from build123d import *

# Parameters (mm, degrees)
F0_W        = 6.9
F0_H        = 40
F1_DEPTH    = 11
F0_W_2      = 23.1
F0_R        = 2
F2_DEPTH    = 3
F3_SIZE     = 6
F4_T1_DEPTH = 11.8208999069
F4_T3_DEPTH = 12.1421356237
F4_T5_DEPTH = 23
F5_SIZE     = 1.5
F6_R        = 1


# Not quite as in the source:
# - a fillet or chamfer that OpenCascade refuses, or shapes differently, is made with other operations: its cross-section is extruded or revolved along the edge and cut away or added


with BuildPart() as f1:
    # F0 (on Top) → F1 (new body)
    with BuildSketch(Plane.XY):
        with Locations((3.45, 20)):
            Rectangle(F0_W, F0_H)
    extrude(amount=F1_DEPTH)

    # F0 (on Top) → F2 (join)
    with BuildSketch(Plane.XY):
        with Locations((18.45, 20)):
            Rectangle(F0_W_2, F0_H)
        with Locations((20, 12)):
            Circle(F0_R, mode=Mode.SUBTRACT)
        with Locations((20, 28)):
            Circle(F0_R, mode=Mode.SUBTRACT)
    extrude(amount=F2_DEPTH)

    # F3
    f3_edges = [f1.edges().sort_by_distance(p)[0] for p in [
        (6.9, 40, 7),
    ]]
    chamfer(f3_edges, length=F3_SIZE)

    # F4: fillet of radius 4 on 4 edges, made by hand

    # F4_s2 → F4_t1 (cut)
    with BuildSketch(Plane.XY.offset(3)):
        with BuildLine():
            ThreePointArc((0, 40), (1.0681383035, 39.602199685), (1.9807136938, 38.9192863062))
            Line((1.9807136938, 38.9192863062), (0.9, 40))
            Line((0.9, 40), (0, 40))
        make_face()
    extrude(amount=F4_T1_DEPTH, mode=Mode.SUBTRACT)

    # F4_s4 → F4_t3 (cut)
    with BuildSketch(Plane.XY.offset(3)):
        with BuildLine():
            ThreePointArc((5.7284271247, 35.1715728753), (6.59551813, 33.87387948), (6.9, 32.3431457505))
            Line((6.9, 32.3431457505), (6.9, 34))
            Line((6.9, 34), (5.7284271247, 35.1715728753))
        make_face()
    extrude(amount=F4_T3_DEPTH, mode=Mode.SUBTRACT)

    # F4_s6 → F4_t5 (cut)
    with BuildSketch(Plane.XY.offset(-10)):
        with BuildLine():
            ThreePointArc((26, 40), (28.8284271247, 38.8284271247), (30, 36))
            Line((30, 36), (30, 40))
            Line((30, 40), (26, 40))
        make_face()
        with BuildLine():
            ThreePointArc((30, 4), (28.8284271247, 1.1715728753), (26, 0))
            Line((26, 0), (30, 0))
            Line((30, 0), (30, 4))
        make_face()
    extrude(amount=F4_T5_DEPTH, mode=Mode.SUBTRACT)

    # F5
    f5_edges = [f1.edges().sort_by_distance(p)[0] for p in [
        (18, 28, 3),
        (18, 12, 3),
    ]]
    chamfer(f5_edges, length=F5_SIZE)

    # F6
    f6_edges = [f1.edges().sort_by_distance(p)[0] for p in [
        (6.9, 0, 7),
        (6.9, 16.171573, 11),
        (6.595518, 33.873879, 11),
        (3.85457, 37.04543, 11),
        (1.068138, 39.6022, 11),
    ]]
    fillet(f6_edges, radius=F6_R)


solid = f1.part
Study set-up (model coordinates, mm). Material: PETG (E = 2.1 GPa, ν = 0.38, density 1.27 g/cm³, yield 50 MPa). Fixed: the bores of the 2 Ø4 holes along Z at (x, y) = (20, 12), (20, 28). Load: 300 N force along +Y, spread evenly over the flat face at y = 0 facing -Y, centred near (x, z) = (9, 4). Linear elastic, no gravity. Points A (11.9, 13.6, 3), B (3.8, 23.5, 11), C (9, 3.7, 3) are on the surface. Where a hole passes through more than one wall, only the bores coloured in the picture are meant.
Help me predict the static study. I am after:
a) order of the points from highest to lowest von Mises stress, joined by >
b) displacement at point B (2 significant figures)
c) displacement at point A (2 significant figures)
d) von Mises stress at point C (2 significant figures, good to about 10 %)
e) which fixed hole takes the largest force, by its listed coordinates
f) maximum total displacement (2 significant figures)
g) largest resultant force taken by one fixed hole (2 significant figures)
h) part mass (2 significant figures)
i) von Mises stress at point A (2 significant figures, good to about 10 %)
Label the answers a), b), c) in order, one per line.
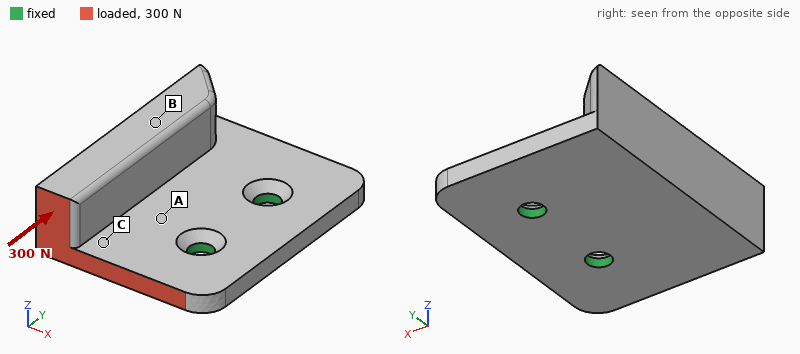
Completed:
a) A > C > B
b) 0.20 mm
c) 0.072 mm
d) 4.7 MPa
e) (20, 12)
f) 0.34 mm
g) 250 N
h) 7.0 g
i) 9.2 MPa
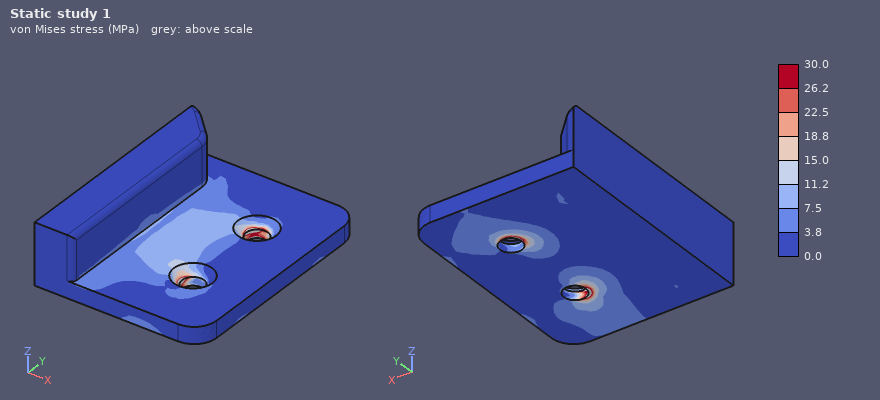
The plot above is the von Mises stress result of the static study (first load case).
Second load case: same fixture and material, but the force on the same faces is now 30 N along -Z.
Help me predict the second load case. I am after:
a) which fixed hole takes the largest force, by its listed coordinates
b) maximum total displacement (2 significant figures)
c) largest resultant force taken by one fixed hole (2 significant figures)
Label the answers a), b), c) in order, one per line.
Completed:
a) (20, 12)
b) 0.54 mm
c) 44 N
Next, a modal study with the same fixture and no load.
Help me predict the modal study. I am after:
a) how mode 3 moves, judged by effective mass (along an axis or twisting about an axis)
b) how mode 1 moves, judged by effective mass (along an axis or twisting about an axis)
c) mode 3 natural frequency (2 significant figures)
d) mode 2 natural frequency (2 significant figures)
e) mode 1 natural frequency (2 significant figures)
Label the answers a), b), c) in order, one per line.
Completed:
a) along Y
b) along Z
c) 3300 Hz
d) 1400 Hz
e) 670 Hz
